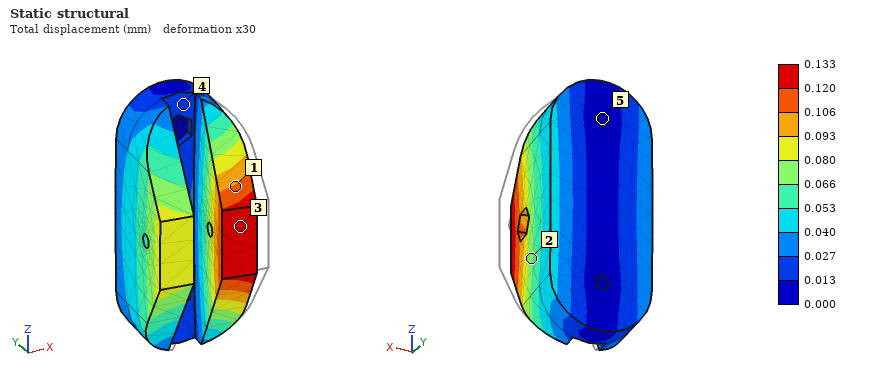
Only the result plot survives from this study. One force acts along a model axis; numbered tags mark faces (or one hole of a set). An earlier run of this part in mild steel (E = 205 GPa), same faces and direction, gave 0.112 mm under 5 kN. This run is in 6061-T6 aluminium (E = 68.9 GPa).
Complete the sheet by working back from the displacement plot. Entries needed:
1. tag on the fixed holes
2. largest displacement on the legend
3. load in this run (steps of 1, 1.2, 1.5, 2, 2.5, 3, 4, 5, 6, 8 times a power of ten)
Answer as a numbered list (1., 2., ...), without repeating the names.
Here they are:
1. 5
2. 0.133 mm
3. 2 kN
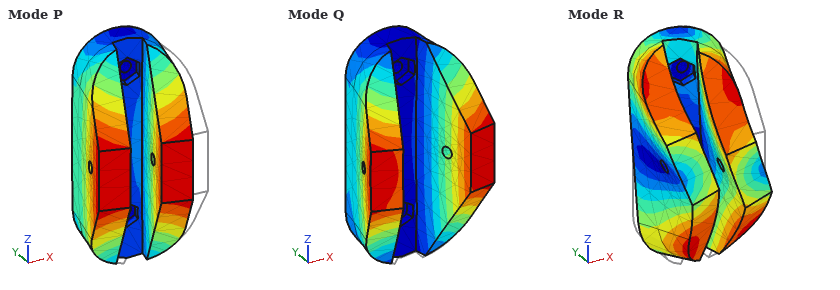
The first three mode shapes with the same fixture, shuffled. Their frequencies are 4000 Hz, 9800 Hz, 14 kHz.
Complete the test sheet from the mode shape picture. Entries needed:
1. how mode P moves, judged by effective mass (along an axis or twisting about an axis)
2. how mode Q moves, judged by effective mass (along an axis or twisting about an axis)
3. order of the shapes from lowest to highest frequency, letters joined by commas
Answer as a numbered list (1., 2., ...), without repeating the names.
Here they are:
1. along X
2. along Y
3. P, Q, R
